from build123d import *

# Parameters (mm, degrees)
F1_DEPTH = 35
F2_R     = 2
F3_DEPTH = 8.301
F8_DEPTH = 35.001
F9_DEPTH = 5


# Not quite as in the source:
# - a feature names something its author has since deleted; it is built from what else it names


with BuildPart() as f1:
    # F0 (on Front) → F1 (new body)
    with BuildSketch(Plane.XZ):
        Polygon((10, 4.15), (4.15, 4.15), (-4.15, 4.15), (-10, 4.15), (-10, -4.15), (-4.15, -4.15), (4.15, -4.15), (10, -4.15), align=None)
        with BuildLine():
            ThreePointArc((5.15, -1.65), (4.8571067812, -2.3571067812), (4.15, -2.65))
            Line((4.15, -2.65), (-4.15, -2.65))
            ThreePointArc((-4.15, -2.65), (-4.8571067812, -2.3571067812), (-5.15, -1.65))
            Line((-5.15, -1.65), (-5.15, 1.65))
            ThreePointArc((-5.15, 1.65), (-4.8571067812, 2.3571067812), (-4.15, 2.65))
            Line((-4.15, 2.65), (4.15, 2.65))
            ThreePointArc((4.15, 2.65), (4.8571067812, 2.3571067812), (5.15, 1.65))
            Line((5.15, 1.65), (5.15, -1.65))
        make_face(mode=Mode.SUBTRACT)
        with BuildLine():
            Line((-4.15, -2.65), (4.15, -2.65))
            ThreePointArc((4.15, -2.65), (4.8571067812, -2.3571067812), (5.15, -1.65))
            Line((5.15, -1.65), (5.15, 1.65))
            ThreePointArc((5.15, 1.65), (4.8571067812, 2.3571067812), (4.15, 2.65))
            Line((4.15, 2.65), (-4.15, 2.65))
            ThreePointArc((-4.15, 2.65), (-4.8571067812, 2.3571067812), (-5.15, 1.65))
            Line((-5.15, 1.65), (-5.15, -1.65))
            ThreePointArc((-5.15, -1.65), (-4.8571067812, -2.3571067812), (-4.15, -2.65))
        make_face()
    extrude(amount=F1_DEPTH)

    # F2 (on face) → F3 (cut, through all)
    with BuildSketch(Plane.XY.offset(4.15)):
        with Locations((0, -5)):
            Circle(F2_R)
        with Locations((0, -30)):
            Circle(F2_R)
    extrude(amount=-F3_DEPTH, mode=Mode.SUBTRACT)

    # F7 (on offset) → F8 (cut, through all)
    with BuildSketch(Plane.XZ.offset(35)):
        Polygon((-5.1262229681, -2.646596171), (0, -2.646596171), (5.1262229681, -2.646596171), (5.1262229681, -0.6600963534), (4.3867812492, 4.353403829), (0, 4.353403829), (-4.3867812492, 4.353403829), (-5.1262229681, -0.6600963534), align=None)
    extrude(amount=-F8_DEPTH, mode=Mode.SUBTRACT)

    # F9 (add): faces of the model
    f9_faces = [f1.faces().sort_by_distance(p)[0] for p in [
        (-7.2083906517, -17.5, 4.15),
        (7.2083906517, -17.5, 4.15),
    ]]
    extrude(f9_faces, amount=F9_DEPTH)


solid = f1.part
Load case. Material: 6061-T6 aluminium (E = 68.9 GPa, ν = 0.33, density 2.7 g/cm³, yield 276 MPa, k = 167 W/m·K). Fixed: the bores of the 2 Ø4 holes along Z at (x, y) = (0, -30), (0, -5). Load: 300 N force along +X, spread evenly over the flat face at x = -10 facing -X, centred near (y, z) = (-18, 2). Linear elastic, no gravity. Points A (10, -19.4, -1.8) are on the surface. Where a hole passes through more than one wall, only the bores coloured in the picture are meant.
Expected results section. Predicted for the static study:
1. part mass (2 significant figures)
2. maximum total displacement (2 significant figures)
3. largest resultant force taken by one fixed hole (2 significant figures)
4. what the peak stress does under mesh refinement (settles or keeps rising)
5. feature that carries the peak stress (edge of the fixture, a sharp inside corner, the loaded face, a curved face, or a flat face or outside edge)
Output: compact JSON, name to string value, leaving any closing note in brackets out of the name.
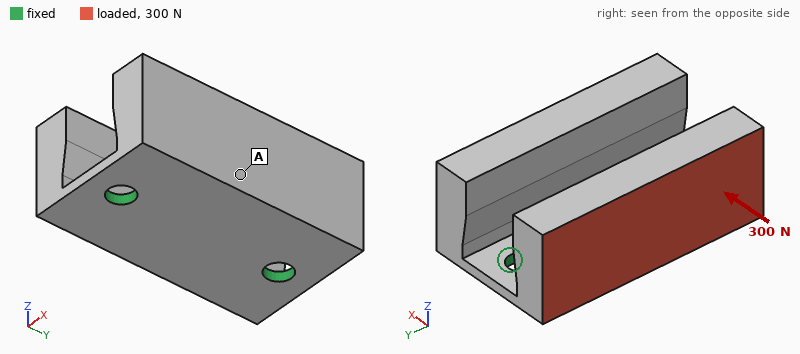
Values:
{"part mass": "15 g", "maximum total displacement": "0.18 mm", "largest resultant force taken by one fixed hole": "150 N", "what the peak stress does under mesh refinement": "keeps rising", "feature that carries the peak stress": "edge of the fixture"}
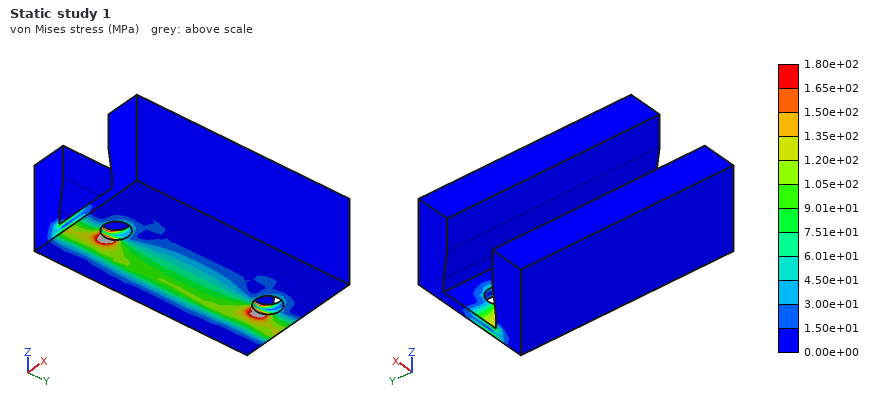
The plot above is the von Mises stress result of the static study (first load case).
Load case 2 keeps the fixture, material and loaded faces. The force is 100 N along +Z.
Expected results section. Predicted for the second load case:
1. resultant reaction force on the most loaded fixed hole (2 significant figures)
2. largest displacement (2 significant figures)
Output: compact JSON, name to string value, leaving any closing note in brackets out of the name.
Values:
{"resultant reaction force on the most loaded fixed hole": "50 N", "largest displacement": "67 µm"}
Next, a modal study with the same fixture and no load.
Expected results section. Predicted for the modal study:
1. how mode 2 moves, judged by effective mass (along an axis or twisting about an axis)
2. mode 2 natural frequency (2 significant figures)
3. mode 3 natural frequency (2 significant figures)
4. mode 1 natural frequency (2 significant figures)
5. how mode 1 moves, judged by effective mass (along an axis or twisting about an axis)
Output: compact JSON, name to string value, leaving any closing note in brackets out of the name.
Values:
{"how mode 2 moves, judged by effective mass": "along Z", "mode 2 natural frequency": "2800 Hz", "mode 3 natural frequency": "9900 Hz", "mode 1 natural frequency": "2700 Hz", "how mode 1 moves, judged by effective mass": "along X"}
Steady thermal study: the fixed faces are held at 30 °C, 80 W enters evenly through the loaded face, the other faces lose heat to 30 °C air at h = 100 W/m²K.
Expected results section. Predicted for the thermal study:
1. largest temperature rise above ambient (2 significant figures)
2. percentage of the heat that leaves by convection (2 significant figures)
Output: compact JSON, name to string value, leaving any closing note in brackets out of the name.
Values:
{"largest temperature rise above ambient": "76 K", "percentage of the heat that leaves by convection": "12 %"}
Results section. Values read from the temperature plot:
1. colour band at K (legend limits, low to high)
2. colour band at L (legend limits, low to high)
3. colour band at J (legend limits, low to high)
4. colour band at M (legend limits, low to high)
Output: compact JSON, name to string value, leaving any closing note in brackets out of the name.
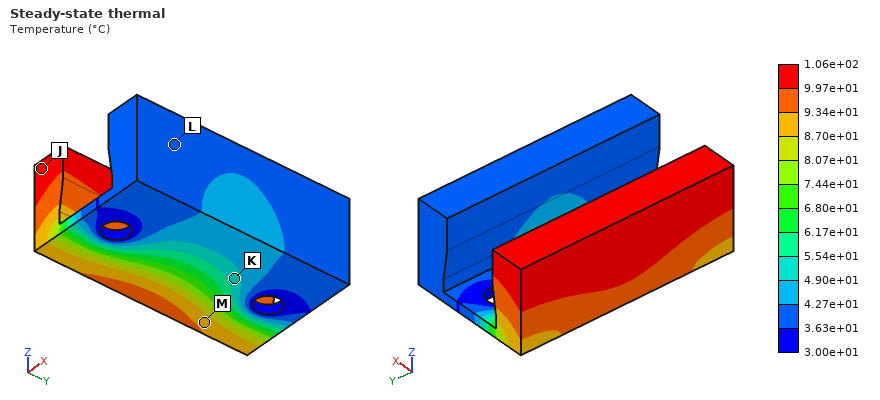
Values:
{"colour band at K": "4.90e+01 to 5.54e+01 °C", "colour band at L": "3.63e+01 to 4.27e+01 °C", "colour band at J": "9.97e+01 to 1.06e+02 °C", "colour band at M": "8.70e+01 to 9.34e+01 °C"}
